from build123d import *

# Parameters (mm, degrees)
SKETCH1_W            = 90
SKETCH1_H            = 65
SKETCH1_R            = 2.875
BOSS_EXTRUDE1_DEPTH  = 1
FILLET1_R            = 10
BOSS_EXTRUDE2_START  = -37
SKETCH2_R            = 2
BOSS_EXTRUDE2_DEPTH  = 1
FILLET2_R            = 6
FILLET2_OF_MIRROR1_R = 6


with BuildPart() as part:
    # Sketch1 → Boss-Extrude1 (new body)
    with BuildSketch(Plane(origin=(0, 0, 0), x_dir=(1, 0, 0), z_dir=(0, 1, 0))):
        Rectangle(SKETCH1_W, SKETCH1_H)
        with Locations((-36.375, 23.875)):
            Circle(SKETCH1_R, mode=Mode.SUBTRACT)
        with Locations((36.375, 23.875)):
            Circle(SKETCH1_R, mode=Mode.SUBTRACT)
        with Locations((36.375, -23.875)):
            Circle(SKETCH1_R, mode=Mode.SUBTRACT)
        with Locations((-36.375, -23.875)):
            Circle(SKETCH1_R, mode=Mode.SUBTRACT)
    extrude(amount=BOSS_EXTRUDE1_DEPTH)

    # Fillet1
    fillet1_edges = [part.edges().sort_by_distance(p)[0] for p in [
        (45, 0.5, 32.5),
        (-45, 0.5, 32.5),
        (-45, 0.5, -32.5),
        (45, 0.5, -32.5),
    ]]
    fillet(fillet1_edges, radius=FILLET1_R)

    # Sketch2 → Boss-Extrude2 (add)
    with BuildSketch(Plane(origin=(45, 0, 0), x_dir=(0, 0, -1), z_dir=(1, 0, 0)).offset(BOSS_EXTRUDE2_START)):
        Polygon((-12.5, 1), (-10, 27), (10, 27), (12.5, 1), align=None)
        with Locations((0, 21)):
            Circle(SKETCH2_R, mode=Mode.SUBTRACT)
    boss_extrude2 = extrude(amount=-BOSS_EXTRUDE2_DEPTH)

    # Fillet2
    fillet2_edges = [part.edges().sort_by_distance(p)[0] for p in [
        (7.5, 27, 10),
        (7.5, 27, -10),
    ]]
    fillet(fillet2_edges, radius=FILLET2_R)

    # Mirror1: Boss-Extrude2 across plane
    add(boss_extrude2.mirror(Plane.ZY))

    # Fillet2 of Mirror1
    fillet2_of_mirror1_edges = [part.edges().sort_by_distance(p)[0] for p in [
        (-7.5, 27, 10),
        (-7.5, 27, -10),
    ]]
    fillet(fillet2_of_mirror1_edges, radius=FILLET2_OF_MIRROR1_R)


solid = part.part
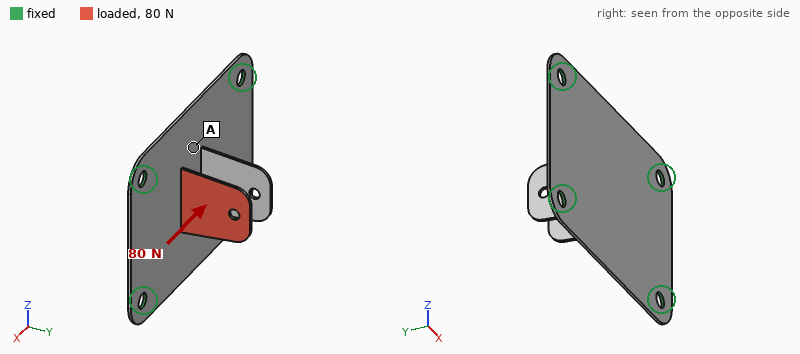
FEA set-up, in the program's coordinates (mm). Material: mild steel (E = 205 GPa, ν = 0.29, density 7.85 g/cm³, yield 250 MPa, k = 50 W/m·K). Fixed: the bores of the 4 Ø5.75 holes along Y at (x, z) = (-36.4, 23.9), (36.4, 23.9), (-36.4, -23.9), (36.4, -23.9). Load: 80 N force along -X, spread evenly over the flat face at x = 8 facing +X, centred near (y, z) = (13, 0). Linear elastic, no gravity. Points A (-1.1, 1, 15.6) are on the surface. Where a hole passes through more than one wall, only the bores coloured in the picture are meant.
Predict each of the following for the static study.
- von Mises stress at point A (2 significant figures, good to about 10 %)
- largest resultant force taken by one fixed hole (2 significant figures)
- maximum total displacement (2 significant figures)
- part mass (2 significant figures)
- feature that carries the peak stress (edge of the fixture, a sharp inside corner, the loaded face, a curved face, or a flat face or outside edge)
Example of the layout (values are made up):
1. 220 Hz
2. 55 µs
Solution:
1. 32 MPa
2. 26 N
3. 0.56 mm
4. 53 g
5. the loaded face
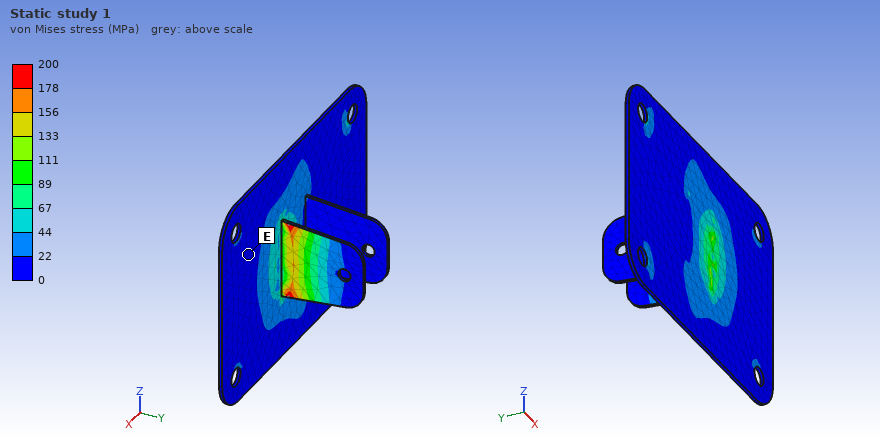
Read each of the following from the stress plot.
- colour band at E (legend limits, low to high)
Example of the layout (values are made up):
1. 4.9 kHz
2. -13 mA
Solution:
1. 0 to 22 MPa
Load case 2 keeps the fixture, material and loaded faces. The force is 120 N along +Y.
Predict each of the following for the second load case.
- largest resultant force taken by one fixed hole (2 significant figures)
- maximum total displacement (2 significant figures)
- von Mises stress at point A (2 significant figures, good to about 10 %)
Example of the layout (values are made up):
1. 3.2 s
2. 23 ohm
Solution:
1. 39 N
2. 0.24 mm
3. 58 MPa
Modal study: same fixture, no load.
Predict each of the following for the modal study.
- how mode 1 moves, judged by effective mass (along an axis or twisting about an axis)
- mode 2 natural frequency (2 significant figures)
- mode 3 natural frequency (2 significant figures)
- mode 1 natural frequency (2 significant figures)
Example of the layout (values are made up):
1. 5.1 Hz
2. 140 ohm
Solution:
1. along Y
2. 1100 Hz
3. 1100 Hz
4. 770 Hz
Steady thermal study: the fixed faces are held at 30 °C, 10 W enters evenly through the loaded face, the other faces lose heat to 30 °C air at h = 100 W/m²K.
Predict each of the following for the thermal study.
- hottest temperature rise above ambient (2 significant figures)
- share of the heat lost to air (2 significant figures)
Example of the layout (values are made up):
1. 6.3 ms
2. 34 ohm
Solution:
1. 81 K
2. 92 %
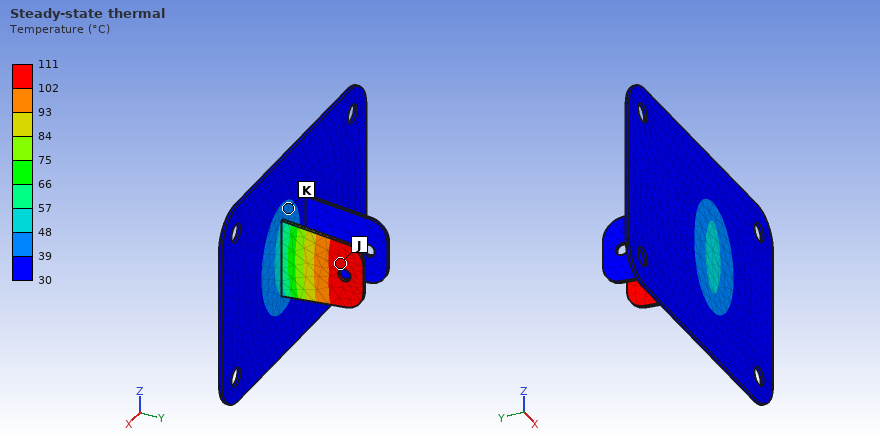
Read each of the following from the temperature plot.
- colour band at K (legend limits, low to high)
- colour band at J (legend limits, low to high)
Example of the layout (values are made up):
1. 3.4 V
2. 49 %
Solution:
1. 39 to 48 °C
2. 102 to 111 °C
